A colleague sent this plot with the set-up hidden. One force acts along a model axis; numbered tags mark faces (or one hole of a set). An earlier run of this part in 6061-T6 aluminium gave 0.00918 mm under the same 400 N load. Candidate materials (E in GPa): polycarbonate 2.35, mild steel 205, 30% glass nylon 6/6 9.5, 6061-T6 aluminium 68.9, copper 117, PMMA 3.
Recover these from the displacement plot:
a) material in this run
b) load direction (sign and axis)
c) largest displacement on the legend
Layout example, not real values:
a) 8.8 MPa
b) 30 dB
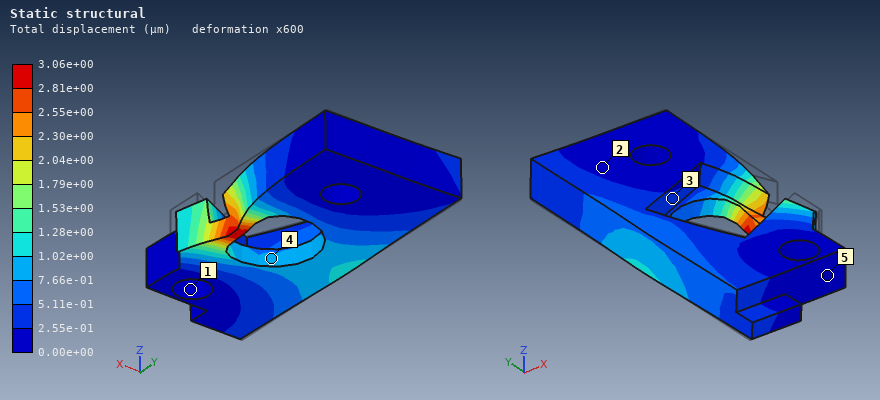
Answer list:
a) mild steel
b) -X
c) 3.06e+00 µm
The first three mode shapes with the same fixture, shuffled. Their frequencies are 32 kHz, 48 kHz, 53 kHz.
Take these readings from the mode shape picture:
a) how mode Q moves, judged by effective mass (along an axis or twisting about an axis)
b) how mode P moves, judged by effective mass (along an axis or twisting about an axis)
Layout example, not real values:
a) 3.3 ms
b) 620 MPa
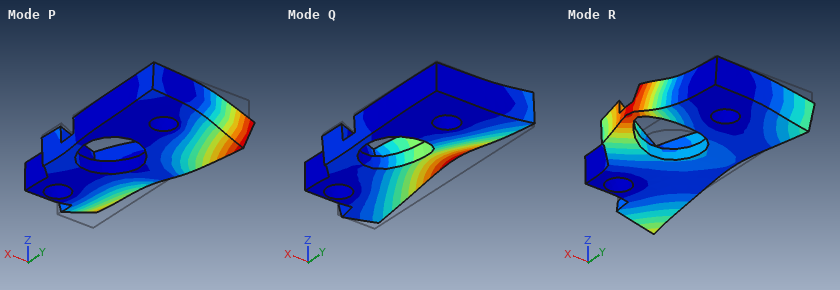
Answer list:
a) along Z
b) twisting about X
